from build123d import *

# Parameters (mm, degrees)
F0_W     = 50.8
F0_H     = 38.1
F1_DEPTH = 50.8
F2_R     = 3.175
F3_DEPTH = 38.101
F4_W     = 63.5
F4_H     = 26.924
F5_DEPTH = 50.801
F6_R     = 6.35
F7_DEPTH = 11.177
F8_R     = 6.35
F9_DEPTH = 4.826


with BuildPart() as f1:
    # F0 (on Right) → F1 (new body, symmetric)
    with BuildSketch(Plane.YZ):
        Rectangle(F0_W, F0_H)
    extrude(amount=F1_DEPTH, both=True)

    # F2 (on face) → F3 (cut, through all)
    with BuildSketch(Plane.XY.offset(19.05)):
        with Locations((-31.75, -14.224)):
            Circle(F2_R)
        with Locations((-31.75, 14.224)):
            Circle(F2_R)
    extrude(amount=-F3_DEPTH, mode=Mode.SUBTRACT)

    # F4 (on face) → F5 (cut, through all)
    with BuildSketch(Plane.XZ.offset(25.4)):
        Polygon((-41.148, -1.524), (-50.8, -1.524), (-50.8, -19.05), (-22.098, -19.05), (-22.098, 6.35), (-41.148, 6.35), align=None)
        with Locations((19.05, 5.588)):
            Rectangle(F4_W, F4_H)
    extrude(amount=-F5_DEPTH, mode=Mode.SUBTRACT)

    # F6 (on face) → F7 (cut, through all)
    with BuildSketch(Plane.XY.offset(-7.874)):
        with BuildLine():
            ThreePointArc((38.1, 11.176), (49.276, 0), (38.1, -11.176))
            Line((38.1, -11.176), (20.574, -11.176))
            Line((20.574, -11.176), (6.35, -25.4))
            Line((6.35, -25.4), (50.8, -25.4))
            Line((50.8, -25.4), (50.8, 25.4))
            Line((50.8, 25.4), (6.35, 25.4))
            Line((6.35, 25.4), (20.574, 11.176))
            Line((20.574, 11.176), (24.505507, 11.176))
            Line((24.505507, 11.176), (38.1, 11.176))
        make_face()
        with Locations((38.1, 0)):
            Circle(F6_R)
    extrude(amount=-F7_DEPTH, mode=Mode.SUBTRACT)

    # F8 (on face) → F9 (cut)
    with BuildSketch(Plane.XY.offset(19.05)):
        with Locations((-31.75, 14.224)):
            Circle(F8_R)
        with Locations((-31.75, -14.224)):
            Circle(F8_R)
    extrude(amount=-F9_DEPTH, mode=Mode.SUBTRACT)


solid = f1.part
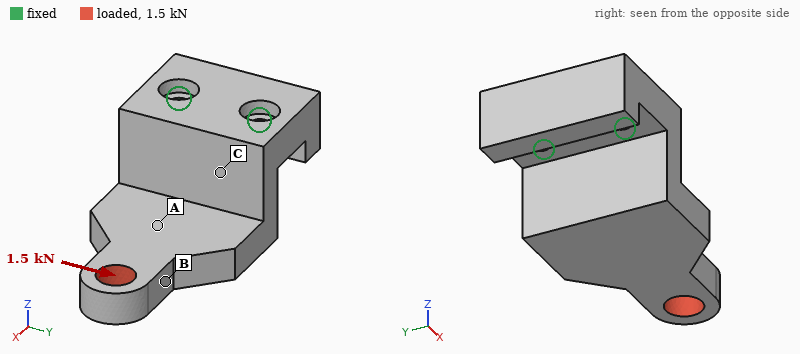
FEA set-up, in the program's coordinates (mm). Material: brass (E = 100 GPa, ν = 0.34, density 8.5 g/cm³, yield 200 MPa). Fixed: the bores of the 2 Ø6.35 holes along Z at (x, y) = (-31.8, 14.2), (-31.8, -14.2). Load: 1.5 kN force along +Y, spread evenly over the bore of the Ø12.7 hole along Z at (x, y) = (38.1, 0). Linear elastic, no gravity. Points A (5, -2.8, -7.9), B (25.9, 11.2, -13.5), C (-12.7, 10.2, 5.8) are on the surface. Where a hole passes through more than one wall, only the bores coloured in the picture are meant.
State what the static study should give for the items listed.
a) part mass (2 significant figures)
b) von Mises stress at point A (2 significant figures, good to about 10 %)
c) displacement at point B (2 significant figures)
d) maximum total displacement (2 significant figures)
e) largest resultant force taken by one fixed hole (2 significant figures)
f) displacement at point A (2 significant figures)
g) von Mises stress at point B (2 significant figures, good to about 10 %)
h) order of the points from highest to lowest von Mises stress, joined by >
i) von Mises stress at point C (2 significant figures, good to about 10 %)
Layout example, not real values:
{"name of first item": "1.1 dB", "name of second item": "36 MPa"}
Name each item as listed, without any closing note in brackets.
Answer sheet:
{"part mass": "520 g", "von Mises stress at point A": "11 MPa", "displacement at point B": "0.089 mm", "maximum total displacement": "0.15 mm", "largest resultant force taken by one fixed hole": "3.6 kN", "displacement at point A": "0.046 mm", "von Mises stress at point B": "28 MPa", "order of the points from highest to lowest von Mises stress, joined by >": "C > B > A", "von Mises stress at point C": "44 MPa"}
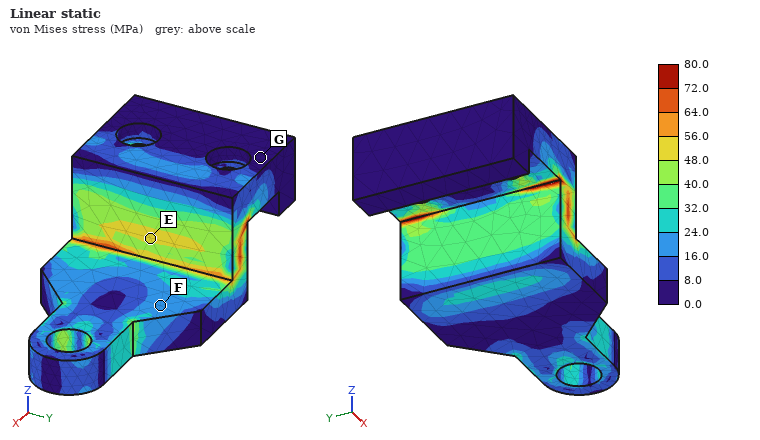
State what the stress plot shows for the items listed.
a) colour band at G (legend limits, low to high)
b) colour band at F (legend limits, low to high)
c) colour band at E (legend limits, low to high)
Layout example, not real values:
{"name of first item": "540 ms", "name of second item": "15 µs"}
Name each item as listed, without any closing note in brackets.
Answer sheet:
{"colour band at G": "0.0 to 8.0 MPa", "colour band at F": "16.0 to 24.0 MPa", "colour band at E": "48.0 to 56.0 MPa"}
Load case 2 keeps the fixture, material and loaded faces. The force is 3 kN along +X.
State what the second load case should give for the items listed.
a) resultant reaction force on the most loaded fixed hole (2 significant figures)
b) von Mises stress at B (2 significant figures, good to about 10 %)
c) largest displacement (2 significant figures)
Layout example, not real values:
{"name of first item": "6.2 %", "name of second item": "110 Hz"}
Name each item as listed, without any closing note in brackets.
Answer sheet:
{"resultant reaction force on the most loaded fixed hole": "1.6 kN", "von Mises stress at B": "20 MPa", "largest displacement": "0.34 mm"}
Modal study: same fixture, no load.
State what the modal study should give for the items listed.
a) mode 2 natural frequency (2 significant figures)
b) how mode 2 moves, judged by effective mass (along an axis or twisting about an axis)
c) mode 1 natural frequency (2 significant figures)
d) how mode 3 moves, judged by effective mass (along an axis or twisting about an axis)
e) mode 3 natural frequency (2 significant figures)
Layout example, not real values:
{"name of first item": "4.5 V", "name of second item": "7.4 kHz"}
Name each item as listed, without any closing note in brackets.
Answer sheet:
{"mode 2 natural frequency": "2200 Hz", "how mode 2 moves, judged by effective mass": "along Y", "mode 1 natural frequency": "930 Hz", "how mode 3 moves, judged by effective mass": "along X", "mode 3 natural frequency": "3400 Hz"}
